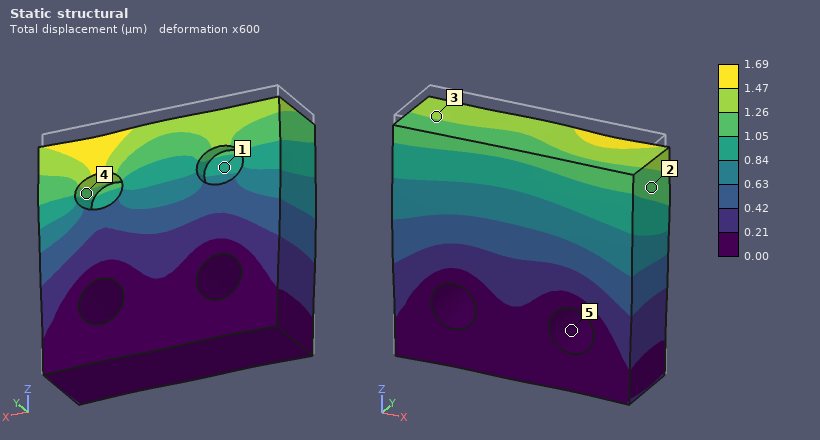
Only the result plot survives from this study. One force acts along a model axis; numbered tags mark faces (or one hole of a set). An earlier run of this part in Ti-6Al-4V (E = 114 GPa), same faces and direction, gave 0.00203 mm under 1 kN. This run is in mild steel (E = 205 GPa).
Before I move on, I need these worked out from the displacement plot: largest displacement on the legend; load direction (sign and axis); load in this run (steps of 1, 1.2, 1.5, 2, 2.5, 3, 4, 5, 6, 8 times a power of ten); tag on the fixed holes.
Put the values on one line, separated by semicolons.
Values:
1.69 µm; -Z; 1.5 kN; 5
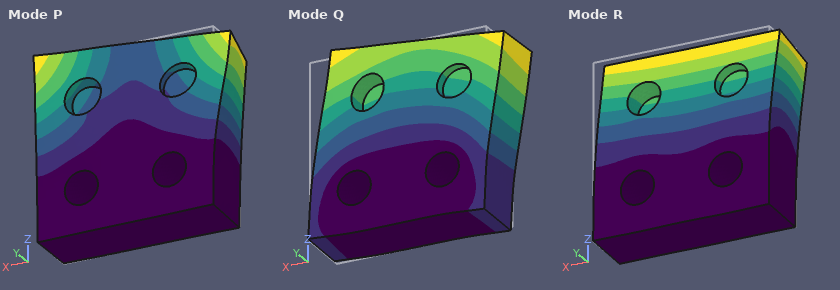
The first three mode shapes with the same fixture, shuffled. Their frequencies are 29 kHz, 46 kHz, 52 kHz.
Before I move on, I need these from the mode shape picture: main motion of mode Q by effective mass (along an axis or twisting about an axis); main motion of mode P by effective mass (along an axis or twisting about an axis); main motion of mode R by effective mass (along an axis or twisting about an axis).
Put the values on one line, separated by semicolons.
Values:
along X; twisting about Z; along Y
